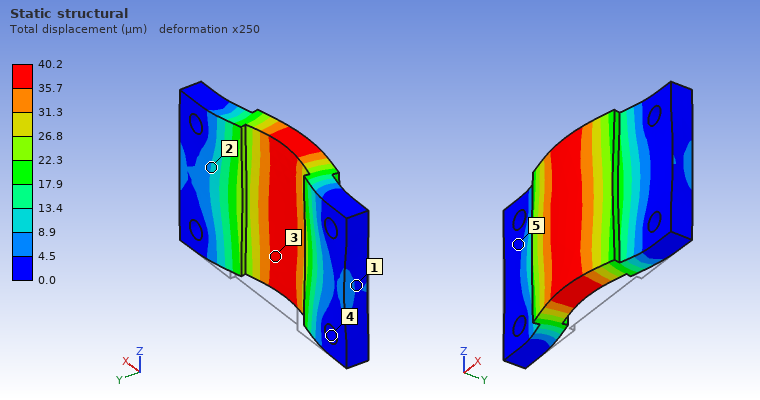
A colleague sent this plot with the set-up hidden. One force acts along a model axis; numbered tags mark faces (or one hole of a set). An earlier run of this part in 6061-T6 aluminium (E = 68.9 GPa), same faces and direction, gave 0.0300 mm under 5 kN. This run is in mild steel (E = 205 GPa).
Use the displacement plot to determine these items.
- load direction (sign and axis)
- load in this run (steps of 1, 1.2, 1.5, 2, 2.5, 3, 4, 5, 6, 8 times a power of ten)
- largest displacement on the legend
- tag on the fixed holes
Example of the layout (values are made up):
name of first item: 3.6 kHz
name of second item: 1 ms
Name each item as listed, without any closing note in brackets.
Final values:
load direction: -Y
load in this run: 20 kN
largest displacement on the legend: 40.2 µm
tag on the fixed holes: 4
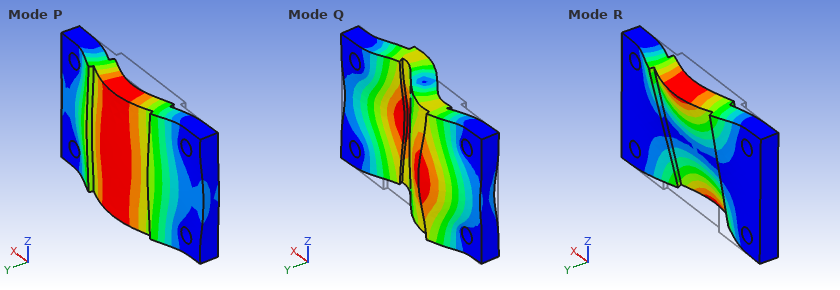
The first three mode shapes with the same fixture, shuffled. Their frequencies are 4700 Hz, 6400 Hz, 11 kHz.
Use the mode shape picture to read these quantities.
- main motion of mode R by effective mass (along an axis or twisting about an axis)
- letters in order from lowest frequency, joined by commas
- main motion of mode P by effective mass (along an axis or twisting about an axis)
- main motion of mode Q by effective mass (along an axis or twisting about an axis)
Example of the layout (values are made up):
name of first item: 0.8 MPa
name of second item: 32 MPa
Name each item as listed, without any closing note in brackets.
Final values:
main motion of mode R by effective mass: twisting about X
letters in order from lowest frequency, joined by commas: P, R, Q
main motion of mode P by effective mass: along Y
main motion of mode Q by effective mass: twisting about Z
